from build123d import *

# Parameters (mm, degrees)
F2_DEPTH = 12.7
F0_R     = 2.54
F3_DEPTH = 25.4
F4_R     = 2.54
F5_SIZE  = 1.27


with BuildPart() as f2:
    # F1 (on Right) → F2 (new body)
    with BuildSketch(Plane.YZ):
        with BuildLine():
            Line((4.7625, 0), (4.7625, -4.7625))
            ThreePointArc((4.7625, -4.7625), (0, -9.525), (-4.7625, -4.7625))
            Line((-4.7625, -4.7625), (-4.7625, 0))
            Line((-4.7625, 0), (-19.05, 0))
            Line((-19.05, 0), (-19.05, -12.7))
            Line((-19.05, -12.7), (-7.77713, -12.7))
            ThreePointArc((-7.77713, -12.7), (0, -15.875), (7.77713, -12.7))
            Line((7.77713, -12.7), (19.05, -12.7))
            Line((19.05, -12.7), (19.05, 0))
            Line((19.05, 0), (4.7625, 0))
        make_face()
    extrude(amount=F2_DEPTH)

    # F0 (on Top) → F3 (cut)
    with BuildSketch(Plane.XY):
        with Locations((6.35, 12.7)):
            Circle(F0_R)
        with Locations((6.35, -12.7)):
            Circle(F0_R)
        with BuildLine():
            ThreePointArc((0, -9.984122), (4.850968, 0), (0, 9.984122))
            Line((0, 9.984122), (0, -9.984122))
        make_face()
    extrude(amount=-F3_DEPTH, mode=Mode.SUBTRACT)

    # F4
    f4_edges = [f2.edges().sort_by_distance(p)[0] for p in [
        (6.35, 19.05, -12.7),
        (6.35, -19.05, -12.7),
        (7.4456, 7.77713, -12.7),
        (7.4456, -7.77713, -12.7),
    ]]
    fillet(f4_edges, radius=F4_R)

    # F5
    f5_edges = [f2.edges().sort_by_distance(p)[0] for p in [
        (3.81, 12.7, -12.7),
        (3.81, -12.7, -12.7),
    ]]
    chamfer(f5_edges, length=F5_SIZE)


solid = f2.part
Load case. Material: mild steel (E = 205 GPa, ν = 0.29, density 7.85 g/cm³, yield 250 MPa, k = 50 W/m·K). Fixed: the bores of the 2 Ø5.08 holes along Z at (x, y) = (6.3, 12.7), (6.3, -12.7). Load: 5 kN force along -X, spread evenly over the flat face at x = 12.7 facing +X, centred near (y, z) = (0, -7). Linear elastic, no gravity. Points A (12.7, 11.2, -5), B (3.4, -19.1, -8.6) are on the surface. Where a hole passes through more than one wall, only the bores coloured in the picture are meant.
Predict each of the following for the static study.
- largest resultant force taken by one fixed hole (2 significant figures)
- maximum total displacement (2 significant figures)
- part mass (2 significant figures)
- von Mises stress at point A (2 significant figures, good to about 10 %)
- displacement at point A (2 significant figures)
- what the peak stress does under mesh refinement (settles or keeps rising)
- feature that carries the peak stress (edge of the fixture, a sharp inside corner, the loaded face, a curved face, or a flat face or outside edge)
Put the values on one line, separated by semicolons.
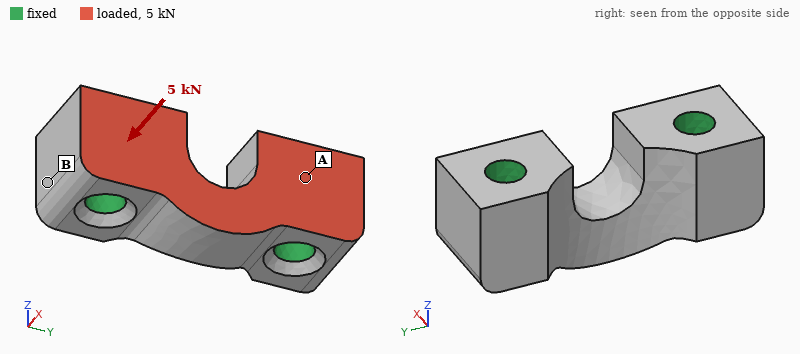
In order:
2.5 kN; 3.1 µm; 34 g; 23 MPa; 0.55 µm; keeps rising; edge of the fixture
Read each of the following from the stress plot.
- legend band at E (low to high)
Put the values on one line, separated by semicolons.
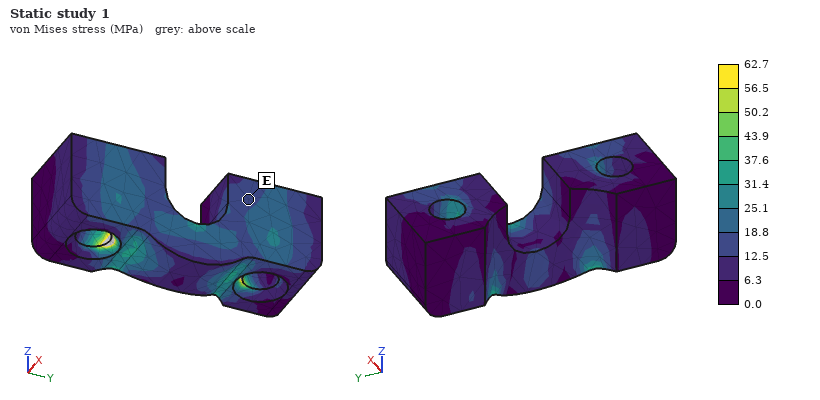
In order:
12.5 to 18.8 MPa
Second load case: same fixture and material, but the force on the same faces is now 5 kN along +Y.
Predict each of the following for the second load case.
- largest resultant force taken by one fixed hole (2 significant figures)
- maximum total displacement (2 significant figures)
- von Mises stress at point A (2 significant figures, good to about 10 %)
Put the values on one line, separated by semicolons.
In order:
2.6 kN; 2.2 µm; 21 MPa
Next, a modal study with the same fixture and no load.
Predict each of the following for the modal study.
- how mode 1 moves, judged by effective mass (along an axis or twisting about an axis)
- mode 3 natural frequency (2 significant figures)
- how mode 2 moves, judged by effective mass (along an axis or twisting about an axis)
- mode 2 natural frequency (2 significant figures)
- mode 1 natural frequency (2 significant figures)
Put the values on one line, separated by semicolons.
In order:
along X; 80 kHz; along Z; 70 kHz; 48 kHz
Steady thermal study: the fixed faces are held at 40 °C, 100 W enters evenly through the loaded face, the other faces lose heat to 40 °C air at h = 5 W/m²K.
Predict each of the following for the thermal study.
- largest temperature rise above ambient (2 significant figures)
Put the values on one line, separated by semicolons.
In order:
52 K
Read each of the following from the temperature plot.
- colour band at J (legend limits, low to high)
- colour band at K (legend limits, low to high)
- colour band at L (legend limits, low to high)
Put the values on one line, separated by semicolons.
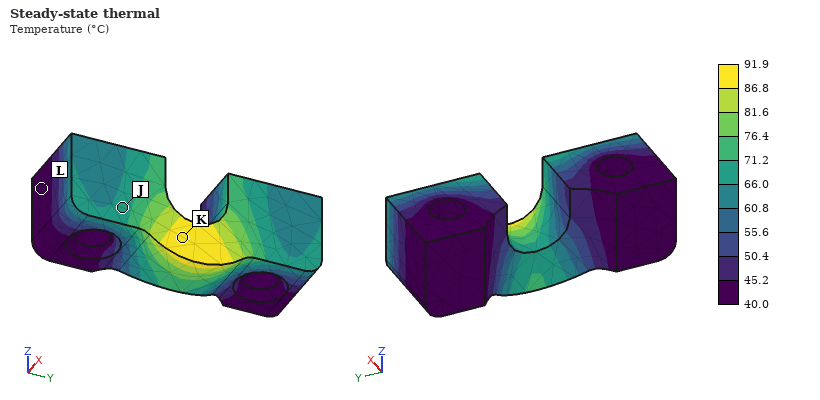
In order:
66.0 to 71.2 °C; 86.8 to 91.9 °C; 40.0 to 45.2 °C
